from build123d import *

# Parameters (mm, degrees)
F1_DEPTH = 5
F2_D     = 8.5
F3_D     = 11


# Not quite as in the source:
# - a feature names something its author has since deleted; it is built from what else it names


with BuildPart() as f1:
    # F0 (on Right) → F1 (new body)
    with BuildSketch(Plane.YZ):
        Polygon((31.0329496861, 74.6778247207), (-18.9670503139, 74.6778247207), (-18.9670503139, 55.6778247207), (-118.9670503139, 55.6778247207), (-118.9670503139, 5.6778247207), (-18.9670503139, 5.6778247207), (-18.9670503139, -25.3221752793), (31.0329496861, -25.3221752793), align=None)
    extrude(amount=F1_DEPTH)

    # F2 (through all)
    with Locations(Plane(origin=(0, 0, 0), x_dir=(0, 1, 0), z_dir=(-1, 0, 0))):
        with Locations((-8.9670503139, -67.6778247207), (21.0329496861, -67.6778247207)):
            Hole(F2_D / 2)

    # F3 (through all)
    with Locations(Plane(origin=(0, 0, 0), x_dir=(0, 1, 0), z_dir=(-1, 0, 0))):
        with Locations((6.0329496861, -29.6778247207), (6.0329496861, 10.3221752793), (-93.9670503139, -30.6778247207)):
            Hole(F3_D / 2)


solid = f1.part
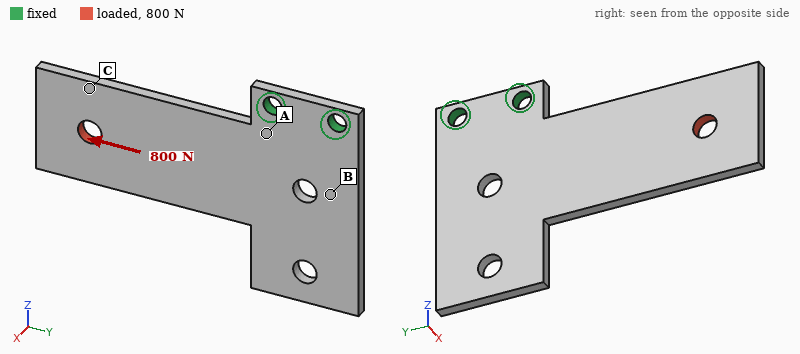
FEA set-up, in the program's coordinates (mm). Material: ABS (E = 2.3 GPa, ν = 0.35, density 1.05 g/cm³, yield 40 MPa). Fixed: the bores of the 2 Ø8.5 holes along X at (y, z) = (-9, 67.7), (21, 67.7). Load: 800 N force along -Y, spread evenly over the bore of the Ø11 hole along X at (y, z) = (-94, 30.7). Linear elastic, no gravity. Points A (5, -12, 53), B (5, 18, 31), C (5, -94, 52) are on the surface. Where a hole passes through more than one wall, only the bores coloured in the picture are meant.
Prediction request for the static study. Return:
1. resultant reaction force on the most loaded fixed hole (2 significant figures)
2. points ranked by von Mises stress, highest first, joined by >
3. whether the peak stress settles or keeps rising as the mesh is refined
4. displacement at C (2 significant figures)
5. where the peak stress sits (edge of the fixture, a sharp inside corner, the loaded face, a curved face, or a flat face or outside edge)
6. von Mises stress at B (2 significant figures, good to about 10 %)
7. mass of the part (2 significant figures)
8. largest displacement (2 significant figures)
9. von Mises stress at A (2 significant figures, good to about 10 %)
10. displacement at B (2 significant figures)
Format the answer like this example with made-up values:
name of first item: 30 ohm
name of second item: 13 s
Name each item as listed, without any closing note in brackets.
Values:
resultant reaction force on the most loaded fixed hole: 890 N
points ranked by von Mises stress, highest first, joined by >: A > B > C
whether the peak stress settles or keeps rising as the mesh is refined: keeps rising
displacement at C: 0.72 mm
where the peak stress sits: edge of the fixture
von Mises stress at B: 5.0 MPa
mass of the part: 50 g
largest displacement: 1.0 mm
von Mises stress at A: 8.9 MPa
displacement at B: 0.25 mm
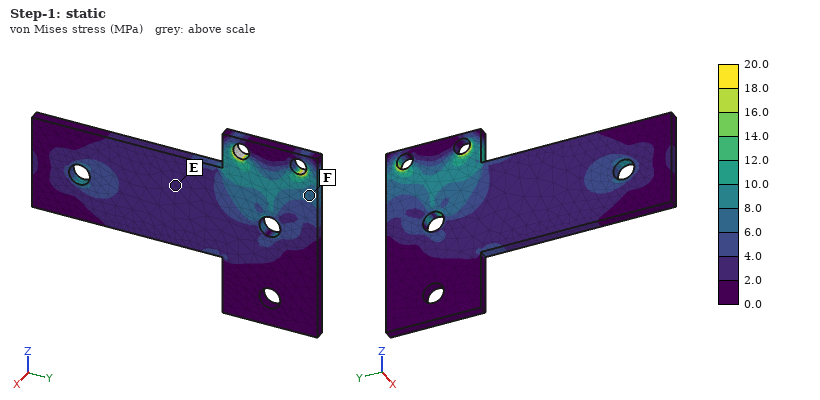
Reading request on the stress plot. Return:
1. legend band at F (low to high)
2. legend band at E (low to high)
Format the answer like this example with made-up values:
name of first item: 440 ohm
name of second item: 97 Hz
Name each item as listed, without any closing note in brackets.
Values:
legend band at F: 6.0 to 8.0 MPa
legend band at E: 2.0 to 4.0 MPa
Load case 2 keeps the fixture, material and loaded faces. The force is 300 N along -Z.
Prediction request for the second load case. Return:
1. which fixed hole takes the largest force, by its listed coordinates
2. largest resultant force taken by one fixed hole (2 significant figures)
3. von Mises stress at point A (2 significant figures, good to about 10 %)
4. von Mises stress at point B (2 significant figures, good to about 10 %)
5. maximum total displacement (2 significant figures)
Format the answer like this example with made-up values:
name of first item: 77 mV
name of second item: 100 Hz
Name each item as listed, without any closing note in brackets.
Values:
which fixed hole takes the largest force, by its listed coordinates: (-9, 67.7)
largest resultant force taken by one fixed hole: 1.0 kN
von Mises stress at point A: 8.1 MPa
von Mises stress at point B: 7.4 MPa
maximum total displacement: 2.1 mm
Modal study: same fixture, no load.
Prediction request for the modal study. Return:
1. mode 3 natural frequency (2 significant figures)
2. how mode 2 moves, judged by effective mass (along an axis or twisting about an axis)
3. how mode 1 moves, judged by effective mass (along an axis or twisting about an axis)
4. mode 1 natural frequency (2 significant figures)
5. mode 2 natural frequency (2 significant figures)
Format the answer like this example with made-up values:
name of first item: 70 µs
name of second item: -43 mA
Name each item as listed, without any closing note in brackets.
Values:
mode 3 natural frequency: 390 Hz
how mode 2 moves, judged by effective mass: along X
how mode 1 moves, judged by effective mass: along X
mode 1 natural frequency: 78 Hz
mode 2 natural frequency: 150 Hz
